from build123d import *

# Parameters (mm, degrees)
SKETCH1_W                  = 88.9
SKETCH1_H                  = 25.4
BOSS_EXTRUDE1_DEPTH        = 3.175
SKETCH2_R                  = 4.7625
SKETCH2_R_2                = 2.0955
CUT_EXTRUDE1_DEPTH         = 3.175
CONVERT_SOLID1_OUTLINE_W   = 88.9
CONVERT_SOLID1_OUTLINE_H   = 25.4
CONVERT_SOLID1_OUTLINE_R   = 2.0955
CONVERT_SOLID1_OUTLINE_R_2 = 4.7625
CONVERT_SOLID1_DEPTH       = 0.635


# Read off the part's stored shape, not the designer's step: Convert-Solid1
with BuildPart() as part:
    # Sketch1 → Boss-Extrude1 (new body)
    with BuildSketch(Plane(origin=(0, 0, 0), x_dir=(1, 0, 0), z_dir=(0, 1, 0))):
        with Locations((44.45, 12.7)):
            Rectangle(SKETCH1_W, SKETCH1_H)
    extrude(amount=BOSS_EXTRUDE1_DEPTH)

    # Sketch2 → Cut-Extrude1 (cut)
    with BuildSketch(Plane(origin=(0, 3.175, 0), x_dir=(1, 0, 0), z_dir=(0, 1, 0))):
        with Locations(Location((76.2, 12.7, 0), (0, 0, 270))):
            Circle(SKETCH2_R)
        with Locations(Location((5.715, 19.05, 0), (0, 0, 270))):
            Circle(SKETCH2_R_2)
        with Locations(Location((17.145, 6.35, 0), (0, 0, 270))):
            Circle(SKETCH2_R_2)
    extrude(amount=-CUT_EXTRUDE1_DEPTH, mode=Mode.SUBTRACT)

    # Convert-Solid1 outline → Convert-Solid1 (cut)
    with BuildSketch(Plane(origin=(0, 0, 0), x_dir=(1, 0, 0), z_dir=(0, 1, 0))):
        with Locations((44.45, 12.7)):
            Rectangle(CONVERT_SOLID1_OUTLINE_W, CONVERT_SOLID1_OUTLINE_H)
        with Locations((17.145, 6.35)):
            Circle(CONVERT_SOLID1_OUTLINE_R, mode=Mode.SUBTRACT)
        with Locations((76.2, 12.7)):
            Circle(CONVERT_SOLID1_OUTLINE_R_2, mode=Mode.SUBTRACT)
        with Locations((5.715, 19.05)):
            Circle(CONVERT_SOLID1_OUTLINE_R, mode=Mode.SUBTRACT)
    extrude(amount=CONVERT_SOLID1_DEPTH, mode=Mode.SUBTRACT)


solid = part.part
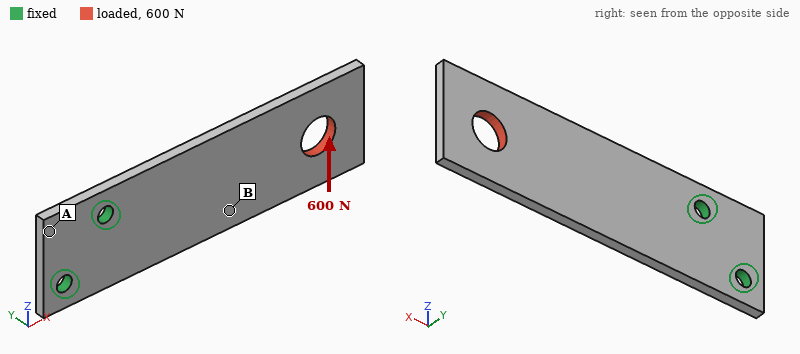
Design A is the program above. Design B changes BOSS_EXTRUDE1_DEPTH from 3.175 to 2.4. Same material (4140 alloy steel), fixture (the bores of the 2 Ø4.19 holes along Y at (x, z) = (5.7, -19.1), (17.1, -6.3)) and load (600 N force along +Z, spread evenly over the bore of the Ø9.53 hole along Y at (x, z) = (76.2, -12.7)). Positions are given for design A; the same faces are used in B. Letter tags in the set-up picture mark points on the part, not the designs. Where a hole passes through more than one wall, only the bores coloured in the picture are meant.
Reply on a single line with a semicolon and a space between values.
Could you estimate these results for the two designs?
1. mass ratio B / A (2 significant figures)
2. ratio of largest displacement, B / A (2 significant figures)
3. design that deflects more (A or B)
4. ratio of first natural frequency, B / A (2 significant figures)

0.69; 1.4; B; 0.70
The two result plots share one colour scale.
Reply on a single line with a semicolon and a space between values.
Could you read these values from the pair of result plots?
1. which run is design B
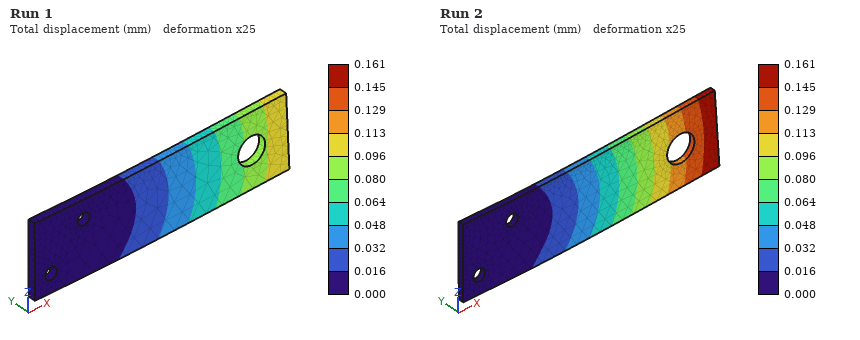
Run 2
